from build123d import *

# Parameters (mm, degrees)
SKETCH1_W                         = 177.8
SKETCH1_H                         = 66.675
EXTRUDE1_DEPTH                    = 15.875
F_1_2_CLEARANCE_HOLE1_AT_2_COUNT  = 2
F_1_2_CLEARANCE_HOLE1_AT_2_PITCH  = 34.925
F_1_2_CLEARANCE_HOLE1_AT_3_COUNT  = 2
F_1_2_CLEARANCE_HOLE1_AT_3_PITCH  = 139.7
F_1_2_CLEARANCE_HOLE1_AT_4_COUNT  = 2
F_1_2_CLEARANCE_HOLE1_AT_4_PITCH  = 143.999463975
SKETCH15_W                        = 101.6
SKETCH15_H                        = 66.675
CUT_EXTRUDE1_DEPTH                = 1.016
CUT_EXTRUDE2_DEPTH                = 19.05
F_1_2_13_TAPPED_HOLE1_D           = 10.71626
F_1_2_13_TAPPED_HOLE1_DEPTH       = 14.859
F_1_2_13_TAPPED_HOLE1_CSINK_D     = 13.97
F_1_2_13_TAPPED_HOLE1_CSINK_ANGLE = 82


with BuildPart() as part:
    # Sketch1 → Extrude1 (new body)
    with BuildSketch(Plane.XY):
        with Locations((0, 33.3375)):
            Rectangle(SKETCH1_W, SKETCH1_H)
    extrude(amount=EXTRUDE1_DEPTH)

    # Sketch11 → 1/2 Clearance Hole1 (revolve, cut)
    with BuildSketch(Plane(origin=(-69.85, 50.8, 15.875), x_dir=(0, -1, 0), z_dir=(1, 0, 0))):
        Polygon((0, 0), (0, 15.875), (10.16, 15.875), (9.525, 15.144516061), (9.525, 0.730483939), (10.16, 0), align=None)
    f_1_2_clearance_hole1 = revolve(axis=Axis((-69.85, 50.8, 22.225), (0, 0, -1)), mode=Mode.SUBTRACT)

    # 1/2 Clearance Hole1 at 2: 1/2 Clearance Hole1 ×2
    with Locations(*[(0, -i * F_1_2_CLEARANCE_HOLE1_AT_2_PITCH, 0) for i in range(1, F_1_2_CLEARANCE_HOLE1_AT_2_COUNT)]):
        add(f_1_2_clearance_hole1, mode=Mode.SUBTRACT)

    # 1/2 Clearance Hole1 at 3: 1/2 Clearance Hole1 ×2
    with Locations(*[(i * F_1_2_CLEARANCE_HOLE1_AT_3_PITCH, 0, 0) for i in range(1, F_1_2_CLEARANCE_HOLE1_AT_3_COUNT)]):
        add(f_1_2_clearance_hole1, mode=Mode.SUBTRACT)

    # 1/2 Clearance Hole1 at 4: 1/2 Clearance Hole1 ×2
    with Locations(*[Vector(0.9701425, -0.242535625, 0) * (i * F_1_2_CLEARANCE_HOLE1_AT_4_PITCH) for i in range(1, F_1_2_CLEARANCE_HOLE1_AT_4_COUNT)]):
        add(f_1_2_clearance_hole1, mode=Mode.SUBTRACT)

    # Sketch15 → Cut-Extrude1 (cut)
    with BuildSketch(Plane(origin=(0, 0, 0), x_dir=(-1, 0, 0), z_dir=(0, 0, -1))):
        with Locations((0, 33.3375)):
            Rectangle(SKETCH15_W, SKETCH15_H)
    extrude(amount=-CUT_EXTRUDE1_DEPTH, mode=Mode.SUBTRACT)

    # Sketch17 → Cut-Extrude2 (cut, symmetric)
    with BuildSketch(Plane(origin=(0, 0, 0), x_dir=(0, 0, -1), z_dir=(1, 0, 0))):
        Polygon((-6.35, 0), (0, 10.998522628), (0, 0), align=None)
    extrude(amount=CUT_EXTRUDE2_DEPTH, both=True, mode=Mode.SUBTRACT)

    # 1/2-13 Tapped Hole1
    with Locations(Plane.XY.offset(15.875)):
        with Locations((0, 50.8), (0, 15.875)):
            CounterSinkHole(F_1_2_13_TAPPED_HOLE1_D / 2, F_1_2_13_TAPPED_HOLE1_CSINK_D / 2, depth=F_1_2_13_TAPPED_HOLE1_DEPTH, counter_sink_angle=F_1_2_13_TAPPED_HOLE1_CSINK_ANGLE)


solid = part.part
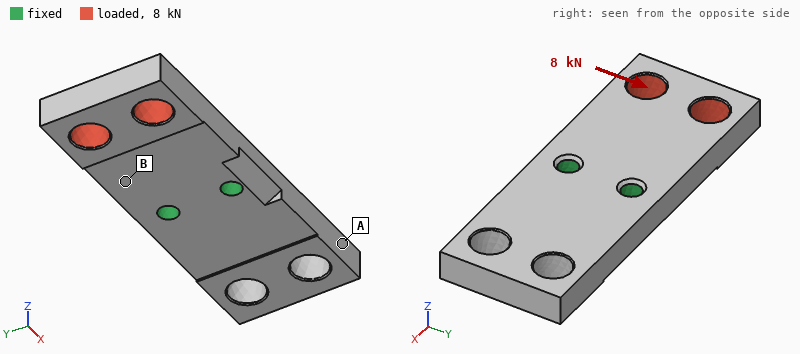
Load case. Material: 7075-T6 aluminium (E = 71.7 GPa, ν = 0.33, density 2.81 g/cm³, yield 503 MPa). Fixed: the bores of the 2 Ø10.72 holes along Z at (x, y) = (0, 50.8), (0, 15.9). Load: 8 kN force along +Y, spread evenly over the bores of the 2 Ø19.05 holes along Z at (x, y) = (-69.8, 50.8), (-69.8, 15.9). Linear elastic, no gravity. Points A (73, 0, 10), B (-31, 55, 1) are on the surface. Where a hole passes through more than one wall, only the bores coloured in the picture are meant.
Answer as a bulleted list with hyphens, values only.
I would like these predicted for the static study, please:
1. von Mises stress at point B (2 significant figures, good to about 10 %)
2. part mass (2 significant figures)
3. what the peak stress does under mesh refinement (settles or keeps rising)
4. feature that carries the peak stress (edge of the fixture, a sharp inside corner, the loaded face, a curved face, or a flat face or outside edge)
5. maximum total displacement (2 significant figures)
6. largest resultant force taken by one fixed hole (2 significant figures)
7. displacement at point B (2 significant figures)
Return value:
- 23 MPa
- 450 g
- keeps rising
- edge of the fixture
- 99 µm
- 14 kN
- 26 µm
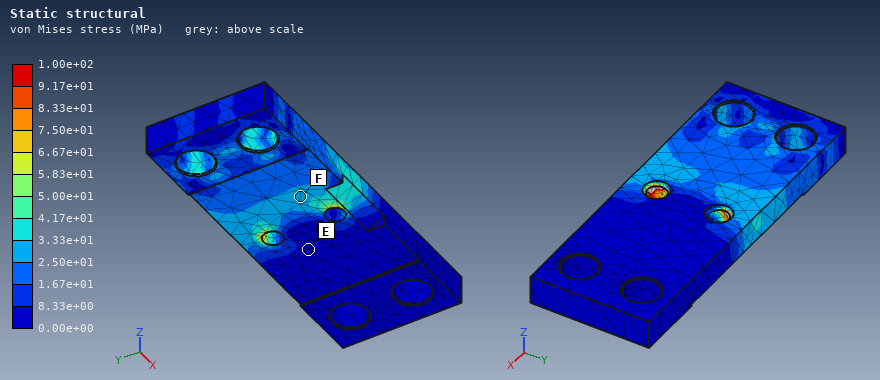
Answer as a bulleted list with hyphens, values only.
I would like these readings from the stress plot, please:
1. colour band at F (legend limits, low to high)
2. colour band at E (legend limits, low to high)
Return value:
- 2.50e+01 to 3.33e+01 MPa
- 0.00e+00 to 8.33e+00 MPa
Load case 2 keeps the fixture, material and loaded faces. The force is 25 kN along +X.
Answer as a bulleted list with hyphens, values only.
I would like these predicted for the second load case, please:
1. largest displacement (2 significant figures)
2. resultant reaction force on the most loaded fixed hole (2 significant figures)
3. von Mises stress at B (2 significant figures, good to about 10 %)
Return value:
- 49 µm
- 13 kN
- 31 MPa
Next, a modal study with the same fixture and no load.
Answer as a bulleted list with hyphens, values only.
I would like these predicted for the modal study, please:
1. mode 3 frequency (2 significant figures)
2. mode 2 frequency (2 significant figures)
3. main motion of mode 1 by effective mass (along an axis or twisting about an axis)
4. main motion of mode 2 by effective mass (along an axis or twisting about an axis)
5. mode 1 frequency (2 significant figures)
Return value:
- 4200 Hz
- 1700 Hz
- twisting about Y
- along Z
- 1600 Hz
